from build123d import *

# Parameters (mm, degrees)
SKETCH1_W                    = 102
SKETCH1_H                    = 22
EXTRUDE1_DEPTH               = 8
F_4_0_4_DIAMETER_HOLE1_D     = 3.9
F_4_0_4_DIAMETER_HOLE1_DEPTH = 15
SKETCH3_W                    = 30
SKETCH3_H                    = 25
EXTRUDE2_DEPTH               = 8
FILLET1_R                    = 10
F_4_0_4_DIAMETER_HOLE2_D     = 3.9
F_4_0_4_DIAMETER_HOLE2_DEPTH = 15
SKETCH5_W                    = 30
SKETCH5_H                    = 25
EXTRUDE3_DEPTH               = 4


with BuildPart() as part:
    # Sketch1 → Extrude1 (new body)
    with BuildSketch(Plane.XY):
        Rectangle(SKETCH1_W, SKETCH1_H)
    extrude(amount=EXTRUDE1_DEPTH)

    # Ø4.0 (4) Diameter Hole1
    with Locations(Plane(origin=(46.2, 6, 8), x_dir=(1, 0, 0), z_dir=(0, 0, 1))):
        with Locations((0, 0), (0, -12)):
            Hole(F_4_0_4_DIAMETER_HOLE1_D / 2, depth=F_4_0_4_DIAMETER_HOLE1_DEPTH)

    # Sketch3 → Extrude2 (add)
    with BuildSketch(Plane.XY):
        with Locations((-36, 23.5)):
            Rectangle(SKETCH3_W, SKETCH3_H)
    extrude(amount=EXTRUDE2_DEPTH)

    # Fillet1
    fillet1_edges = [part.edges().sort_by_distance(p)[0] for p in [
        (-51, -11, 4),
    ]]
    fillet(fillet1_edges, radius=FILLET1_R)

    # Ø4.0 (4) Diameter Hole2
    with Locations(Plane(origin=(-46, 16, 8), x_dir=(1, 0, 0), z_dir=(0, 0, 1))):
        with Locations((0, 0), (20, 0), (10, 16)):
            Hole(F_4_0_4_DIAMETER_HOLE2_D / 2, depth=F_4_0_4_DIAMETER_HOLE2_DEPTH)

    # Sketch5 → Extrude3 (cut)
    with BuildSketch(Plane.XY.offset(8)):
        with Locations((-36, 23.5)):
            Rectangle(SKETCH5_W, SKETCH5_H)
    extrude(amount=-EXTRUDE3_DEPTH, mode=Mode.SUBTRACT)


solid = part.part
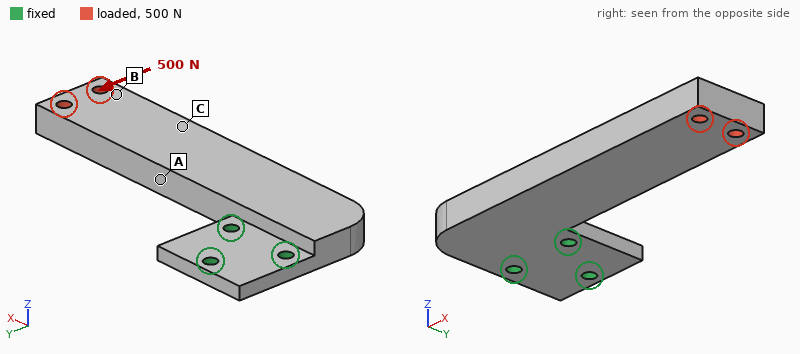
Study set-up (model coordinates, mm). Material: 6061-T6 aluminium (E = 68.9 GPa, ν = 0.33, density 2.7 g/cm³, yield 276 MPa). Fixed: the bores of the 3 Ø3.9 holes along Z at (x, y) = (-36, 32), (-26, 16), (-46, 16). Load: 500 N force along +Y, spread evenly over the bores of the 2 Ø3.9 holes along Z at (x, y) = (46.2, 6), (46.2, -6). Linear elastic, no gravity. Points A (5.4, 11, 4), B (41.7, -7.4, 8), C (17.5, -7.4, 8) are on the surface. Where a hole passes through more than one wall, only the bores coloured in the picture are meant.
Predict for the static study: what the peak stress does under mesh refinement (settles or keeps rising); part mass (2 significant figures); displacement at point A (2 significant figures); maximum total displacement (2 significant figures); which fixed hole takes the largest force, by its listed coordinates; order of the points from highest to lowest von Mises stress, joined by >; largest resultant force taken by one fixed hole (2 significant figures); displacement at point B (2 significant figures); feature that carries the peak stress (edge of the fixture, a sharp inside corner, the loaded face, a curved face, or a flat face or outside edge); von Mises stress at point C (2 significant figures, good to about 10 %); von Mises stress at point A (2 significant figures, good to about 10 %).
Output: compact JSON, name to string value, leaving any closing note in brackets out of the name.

{"what the peak stress does under mesh refinement": "keeps rising", "part mass": "55 g", "displacement at point A": "0.088 mm", "maximum total displacement": "0.27 mm", "which fixed hole takes the largest force, by its listed coordinates": "(-26, 16)", "order of the points from highest to lowest von Mises stress, joined by >": "A > C > B", "largest resultant force taken by one fixed hole": "2.1 kN", "displacement at point B": "0.23 mm", "feature that carries the peak stress": "edge of the fixture", "von Mises stress at point C": "15 MPa", "von Mises stress at point A": "32 MPa"}
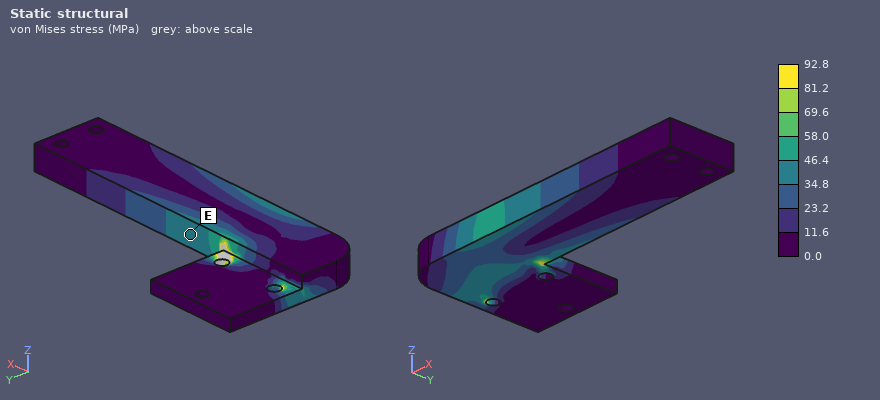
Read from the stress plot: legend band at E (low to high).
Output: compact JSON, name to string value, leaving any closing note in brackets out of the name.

{"legend band at E": "34.8 to 46.4 MPa"}
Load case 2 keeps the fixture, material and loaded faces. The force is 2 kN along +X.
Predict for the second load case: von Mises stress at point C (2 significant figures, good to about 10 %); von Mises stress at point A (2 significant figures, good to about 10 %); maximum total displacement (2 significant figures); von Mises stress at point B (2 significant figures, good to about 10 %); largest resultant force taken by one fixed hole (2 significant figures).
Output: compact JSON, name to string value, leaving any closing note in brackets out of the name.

{"von Mises stress at point C": "11 MPa", "von Mises stress at point A": "11 MPa", "maximum total displacement": "61 µm", "von Mises stress at point B": "13 MPa", "largest resultant force taken by one fixed hole": "1.8 kN"}
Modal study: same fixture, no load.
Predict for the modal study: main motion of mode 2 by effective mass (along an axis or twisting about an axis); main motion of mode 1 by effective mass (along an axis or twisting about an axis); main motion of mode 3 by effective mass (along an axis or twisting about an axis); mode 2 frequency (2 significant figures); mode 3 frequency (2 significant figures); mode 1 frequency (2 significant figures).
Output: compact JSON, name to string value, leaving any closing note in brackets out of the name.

{"main motion of mode 2 by effective mass": "along Y", "main motion of mode 1 by effective mass": "along Z", "main motion of mode 3 by effective mass": "along Z", "mode 2 frequency": "2100 Hz", "mode 3 frequency": "2700 Hz", "mode 1 frequency": "800 Hz"}
